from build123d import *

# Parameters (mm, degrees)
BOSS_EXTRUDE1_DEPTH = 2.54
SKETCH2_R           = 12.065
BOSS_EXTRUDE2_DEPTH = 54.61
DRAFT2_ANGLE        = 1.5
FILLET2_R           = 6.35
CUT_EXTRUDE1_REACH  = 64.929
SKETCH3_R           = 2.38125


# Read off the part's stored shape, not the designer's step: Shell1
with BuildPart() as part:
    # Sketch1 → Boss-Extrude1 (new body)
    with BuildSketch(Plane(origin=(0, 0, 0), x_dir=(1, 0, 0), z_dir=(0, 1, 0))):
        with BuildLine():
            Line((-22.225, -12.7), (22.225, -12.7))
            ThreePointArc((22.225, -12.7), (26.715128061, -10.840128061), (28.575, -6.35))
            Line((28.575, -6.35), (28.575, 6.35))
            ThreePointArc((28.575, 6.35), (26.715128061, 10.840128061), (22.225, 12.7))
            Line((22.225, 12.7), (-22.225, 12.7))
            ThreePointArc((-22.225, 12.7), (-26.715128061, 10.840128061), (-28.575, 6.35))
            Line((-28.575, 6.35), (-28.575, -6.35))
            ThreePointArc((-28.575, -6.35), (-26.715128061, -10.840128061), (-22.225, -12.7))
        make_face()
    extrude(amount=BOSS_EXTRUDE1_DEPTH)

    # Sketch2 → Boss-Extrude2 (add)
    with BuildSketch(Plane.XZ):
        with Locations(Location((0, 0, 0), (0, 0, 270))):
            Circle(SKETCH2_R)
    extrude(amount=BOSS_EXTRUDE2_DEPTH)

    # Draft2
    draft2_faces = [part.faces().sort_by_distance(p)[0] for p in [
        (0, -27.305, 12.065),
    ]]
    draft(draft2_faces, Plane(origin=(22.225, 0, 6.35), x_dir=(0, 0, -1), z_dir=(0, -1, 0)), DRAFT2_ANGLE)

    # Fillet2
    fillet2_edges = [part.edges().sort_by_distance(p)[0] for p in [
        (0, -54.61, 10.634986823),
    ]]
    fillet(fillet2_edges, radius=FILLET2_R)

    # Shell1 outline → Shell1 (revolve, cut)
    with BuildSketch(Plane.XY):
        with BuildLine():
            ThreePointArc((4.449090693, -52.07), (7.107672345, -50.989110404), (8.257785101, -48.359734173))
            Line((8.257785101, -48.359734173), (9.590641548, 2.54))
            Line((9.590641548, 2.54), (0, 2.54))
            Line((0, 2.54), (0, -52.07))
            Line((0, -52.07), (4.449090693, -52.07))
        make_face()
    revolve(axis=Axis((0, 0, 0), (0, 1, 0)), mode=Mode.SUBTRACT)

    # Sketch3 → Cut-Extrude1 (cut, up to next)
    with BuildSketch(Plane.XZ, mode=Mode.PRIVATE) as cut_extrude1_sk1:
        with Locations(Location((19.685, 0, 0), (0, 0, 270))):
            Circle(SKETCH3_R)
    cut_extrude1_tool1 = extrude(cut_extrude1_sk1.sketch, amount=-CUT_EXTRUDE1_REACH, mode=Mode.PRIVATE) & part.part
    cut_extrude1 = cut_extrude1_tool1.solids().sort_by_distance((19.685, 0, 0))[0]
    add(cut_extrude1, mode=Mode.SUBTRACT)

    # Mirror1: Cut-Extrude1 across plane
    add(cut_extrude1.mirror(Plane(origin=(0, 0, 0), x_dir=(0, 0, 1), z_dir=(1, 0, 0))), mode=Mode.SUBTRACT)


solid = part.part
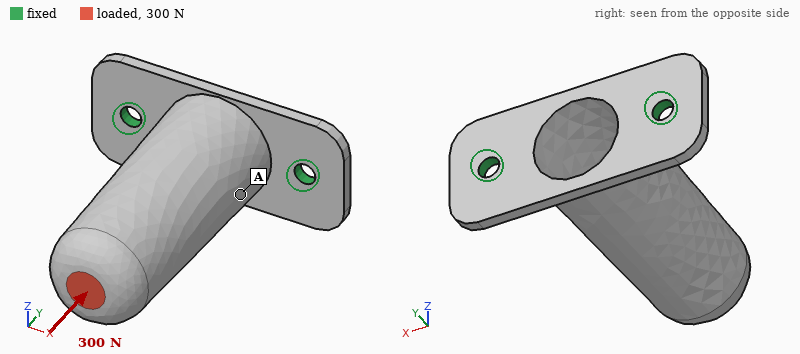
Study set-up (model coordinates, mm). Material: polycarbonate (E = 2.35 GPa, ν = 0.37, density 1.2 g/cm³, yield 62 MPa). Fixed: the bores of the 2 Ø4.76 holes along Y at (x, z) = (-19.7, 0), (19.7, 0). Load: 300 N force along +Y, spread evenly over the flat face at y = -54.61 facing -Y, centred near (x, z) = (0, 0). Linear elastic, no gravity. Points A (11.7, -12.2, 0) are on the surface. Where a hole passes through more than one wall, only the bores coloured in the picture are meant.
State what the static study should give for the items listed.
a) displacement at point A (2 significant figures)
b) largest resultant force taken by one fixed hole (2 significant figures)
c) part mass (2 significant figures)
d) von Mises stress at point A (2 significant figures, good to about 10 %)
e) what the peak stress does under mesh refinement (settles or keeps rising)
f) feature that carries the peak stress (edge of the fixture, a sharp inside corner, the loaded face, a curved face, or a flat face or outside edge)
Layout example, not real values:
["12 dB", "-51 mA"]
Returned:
["0.22 mm", "160 N", "14 g", "3.9 MPa", "keeps rising", "edge of the fixture"]
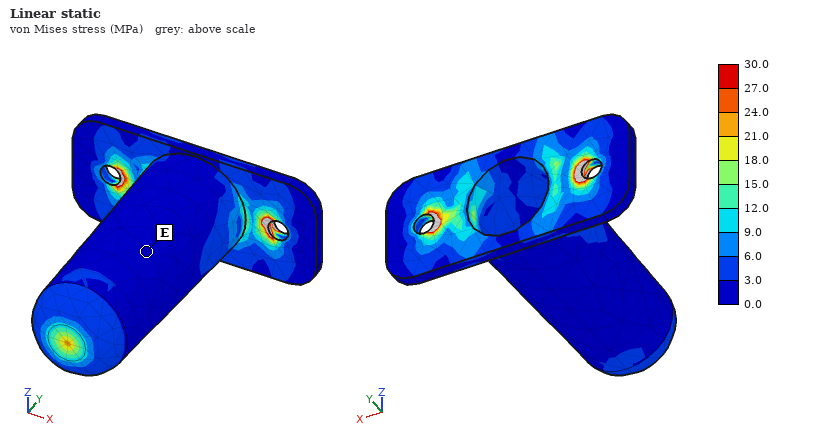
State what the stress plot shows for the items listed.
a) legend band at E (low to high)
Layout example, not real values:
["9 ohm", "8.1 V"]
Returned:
["0.0 to 3.0 MPa"]
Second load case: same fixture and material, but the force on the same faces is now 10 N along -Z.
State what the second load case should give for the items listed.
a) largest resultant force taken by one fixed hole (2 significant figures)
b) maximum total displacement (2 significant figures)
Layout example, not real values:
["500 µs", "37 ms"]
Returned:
["5.0 N", "0.94 mm"]
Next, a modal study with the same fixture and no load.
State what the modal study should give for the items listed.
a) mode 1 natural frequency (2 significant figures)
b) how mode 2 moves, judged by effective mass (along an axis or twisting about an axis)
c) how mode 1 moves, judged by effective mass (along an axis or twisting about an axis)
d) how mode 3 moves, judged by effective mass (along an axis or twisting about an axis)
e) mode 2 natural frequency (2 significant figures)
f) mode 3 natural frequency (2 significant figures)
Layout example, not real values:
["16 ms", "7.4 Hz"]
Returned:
["270 Hz", "along X", "along Z", "along Y", "750 Hz", "1700 Hz"]
